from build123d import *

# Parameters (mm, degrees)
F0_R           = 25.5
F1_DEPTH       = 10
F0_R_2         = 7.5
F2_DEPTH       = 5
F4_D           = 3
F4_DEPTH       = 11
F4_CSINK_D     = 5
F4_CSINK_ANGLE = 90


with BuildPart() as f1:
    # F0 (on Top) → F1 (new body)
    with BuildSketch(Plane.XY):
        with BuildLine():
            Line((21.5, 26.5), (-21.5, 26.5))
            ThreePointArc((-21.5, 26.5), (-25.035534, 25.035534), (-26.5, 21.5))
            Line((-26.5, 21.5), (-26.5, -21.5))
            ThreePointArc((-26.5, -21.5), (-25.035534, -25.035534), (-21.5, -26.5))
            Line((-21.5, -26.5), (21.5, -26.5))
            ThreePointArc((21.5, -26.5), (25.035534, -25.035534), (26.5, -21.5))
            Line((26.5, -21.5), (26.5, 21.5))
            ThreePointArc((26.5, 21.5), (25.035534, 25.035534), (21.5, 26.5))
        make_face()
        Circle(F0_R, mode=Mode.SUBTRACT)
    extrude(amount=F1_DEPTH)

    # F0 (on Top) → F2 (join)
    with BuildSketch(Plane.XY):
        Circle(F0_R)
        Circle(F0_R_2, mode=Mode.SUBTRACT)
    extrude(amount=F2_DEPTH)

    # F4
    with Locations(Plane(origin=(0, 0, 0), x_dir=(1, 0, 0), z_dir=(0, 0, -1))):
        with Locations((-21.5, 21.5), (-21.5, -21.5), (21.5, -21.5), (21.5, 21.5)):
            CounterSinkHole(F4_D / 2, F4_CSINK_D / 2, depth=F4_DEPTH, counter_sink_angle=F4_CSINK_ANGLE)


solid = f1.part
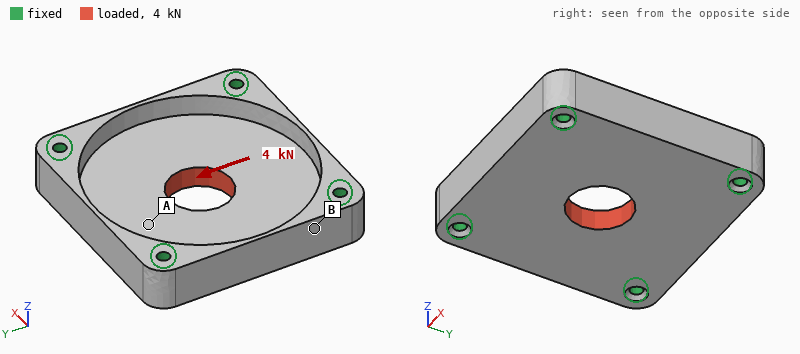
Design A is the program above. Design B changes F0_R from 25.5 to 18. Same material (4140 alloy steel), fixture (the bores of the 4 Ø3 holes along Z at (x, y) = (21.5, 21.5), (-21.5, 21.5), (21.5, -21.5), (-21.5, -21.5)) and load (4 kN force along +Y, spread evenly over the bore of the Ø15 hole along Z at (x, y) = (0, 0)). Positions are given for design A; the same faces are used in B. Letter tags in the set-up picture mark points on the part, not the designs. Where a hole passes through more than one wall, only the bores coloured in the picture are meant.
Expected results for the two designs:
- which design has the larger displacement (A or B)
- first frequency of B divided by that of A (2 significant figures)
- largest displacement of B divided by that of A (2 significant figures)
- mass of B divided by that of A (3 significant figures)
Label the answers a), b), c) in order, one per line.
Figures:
a) A
b) 1.3
c) 0.89
d) 1.31
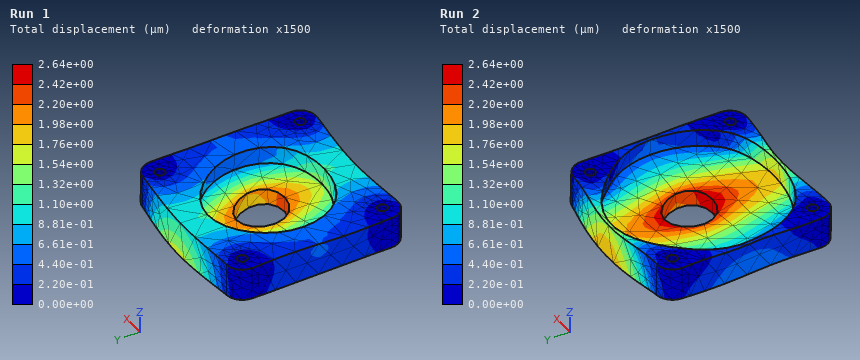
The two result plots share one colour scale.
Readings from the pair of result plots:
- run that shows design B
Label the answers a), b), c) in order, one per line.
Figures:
a) Run 1
